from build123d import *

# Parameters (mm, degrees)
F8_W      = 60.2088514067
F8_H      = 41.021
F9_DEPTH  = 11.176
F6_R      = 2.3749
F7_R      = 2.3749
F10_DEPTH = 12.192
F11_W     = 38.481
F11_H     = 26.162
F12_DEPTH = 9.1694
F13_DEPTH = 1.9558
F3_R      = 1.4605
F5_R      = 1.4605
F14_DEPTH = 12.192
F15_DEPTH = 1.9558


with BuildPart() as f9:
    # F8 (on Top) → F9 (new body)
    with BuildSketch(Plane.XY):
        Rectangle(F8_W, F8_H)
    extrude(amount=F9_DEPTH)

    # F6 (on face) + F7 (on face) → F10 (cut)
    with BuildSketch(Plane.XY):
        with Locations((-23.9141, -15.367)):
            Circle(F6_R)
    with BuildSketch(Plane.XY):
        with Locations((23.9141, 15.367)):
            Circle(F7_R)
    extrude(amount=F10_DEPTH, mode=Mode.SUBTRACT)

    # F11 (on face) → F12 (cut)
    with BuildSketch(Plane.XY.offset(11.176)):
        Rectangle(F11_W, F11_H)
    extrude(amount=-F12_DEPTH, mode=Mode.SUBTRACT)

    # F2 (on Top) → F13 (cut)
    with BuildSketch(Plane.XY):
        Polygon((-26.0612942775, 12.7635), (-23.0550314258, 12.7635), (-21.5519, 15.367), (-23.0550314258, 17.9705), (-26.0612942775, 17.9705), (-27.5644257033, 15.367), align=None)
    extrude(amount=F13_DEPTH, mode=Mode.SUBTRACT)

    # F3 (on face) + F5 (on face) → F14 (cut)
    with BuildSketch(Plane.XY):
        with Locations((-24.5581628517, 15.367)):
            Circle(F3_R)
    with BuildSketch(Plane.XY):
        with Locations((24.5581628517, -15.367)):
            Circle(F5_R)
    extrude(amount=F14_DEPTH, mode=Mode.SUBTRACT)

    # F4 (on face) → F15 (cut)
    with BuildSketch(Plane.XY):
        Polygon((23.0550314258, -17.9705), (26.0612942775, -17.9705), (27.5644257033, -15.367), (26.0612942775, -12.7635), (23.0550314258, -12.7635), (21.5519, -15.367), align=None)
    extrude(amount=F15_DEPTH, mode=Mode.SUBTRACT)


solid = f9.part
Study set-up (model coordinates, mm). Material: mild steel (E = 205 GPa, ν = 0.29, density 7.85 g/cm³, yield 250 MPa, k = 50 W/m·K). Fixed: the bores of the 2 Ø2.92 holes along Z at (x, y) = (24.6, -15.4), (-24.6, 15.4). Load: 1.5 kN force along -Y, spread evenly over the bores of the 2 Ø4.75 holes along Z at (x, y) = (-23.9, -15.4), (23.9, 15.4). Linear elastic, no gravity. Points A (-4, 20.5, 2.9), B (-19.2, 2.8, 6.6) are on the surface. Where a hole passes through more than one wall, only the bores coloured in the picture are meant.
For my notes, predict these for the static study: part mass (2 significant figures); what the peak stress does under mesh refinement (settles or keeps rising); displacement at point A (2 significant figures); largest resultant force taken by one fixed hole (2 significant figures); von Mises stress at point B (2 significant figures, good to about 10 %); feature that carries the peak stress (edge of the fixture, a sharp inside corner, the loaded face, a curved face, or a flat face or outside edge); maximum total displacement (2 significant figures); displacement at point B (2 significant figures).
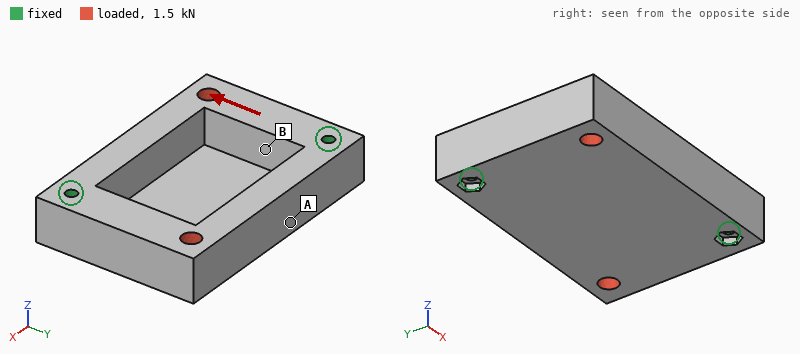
140 g
keeps rising
0.52 µm
750 N
5.6 MPa
edge of the fixture
1.3 µm
0.45 µm
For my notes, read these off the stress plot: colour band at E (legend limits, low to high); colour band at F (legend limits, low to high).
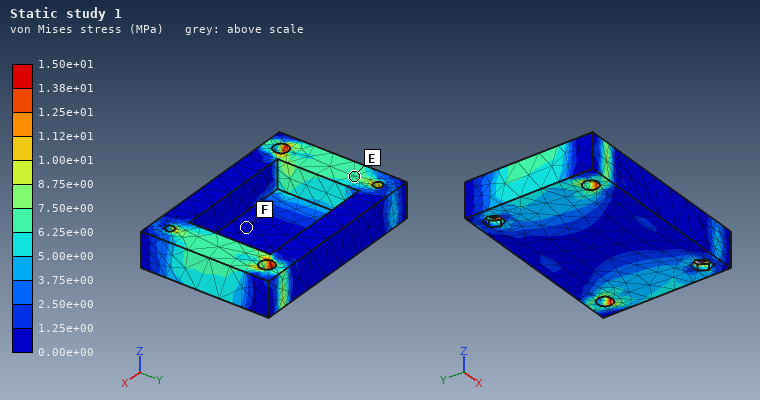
6.25e+00 to 7.50e+00 MPa
0.00e+00 to 1.25e+00 MPa
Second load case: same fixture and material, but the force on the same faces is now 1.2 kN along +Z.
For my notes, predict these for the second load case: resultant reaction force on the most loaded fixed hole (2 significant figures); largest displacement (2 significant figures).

1.0 kN
17 µm
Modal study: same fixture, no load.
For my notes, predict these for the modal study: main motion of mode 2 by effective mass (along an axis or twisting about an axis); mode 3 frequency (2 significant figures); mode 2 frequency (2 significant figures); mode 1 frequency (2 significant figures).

along Z
14 kHz
7200 Hz
5800 Hz
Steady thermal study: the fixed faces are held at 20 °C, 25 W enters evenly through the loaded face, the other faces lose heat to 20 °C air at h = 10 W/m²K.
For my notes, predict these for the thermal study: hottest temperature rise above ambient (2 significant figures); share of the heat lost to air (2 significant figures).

45 K
7.1 %
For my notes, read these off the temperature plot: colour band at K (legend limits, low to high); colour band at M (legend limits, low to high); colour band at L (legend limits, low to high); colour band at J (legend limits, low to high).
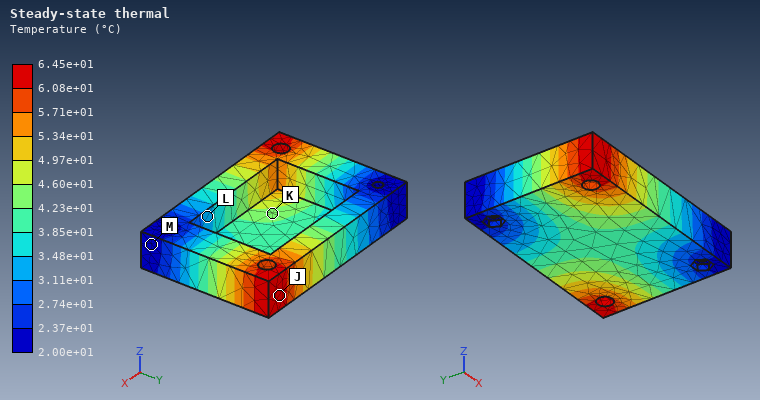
4.23e+01 to 4.60e+01 °C
2.00e+01 to 2.37e+01 °C
3.11e+01 to 3.48e+01 °C
6.08e+01 to 6.45e+01 °C
